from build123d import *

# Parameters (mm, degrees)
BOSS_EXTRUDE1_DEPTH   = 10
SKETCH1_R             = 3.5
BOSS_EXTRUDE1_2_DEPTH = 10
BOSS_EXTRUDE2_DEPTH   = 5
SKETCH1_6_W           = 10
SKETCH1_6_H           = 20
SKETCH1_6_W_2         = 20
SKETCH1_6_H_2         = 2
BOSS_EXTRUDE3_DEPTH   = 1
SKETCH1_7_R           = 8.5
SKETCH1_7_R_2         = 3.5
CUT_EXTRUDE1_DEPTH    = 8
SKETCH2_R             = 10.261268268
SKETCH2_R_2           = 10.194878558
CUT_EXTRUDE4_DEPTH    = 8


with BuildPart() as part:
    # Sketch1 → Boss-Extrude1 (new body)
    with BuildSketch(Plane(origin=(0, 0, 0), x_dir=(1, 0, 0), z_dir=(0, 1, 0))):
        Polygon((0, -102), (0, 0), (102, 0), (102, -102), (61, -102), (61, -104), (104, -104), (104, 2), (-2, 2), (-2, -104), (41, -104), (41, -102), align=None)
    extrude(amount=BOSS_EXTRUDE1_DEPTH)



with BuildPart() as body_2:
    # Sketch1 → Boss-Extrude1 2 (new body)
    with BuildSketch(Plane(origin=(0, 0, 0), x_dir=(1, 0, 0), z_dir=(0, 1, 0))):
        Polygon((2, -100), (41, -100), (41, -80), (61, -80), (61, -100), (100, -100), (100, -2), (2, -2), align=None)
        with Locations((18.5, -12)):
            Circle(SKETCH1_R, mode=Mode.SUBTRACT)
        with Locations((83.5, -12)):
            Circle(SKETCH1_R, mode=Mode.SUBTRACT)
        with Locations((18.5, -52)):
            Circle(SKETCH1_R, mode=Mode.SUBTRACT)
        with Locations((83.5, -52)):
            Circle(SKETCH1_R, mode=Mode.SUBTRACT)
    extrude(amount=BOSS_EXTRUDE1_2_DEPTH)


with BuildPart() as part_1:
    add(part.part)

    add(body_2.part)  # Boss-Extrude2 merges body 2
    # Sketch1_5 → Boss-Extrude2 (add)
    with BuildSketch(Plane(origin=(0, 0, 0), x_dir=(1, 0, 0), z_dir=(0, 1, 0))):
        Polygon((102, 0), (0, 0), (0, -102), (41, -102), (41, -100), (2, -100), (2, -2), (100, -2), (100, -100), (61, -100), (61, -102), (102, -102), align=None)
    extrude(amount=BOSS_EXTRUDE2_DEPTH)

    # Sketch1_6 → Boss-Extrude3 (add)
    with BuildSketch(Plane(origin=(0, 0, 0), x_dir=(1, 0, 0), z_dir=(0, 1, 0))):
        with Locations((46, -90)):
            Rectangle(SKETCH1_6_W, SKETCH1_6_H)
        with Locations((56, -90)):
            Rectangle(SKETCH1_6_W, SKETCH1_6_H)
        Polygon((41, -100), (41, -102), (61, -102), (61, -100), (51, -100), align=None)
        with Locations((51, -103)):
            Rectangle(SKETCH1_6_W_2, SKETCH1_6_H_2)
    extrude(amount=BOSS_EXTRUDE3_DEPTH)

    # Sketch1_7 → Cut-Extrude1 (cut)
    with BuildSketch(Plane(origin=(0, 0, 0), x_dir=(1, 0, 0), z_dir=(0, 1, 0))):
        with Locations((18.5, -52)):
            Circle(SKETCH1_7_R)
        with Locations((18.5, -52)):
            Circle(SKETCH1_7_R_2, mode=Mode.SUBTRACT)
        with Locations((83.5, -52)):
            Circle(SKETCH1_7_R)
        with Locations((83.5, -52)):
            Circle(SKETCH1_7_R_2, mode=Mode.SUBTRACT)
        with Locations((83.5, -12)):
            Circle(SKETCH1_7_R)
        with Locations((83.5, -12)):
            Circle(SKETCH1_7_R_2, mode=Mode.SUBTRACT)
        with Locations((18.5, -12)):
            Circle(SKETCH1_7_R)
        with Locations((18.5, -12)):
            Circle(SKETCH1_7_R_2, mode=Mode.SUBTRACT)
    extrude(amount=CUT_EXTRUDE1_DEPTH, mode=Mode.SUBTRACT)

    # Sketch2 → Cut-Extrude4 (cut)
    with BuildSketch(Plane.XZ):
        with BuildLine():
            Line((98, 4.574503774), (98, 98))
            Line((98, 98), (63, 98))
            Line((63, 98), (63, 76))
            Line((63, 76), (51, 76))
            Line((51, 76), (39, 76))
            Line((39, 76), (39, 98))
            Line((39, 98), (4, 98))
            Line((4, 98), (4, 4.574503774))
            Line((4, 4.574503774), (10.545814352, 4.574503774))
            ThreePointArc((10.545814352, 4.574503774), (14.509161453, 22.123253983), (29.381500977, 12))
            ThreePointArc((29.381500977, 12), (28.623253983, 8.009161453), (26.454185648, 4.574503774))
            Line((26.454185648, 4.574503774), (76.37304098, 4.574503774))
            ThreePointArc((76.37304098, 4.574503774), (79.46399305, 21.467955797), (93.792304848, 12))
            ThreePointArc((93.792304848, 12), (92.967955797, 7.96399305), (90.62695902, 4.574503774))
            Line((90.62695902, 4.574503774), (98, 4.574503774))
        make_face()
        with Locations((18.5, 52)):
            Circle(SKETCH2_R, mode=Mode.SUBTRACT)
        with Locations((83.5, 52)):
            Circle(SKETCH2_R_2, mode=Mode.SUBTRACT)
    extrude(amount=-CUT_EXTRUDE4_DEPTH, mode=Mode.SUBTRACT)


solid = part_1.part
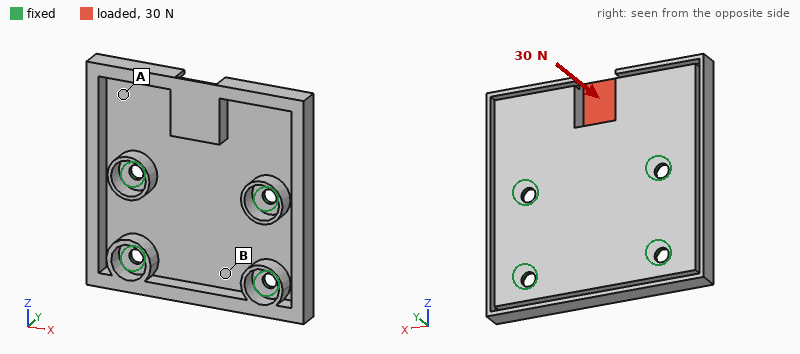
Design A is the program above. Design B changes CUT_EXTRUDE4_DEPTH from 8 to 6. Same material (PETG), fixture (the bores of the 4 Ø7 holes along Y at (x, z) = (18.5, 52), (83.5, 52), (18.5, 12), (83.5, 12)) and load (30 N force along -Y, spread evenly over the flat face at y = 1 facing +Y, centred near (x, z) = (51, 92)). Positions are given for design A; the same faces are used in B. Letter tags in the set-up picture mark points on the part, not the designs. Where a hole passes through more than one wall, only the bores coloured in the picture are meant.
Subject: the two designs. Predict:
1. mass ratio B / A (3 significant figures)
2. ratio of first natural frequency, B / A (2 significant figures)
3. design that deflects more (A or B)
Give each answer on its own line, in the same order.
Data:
1.34
1.3
A
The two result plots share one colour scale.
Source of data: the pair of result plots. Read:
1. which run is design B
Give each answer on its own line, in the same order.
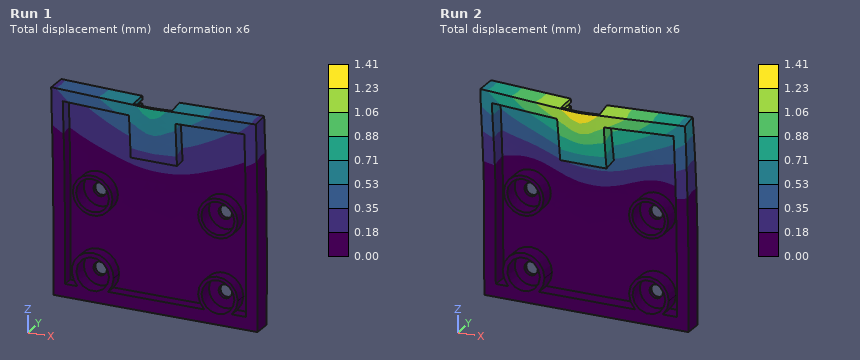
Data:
Run 1
